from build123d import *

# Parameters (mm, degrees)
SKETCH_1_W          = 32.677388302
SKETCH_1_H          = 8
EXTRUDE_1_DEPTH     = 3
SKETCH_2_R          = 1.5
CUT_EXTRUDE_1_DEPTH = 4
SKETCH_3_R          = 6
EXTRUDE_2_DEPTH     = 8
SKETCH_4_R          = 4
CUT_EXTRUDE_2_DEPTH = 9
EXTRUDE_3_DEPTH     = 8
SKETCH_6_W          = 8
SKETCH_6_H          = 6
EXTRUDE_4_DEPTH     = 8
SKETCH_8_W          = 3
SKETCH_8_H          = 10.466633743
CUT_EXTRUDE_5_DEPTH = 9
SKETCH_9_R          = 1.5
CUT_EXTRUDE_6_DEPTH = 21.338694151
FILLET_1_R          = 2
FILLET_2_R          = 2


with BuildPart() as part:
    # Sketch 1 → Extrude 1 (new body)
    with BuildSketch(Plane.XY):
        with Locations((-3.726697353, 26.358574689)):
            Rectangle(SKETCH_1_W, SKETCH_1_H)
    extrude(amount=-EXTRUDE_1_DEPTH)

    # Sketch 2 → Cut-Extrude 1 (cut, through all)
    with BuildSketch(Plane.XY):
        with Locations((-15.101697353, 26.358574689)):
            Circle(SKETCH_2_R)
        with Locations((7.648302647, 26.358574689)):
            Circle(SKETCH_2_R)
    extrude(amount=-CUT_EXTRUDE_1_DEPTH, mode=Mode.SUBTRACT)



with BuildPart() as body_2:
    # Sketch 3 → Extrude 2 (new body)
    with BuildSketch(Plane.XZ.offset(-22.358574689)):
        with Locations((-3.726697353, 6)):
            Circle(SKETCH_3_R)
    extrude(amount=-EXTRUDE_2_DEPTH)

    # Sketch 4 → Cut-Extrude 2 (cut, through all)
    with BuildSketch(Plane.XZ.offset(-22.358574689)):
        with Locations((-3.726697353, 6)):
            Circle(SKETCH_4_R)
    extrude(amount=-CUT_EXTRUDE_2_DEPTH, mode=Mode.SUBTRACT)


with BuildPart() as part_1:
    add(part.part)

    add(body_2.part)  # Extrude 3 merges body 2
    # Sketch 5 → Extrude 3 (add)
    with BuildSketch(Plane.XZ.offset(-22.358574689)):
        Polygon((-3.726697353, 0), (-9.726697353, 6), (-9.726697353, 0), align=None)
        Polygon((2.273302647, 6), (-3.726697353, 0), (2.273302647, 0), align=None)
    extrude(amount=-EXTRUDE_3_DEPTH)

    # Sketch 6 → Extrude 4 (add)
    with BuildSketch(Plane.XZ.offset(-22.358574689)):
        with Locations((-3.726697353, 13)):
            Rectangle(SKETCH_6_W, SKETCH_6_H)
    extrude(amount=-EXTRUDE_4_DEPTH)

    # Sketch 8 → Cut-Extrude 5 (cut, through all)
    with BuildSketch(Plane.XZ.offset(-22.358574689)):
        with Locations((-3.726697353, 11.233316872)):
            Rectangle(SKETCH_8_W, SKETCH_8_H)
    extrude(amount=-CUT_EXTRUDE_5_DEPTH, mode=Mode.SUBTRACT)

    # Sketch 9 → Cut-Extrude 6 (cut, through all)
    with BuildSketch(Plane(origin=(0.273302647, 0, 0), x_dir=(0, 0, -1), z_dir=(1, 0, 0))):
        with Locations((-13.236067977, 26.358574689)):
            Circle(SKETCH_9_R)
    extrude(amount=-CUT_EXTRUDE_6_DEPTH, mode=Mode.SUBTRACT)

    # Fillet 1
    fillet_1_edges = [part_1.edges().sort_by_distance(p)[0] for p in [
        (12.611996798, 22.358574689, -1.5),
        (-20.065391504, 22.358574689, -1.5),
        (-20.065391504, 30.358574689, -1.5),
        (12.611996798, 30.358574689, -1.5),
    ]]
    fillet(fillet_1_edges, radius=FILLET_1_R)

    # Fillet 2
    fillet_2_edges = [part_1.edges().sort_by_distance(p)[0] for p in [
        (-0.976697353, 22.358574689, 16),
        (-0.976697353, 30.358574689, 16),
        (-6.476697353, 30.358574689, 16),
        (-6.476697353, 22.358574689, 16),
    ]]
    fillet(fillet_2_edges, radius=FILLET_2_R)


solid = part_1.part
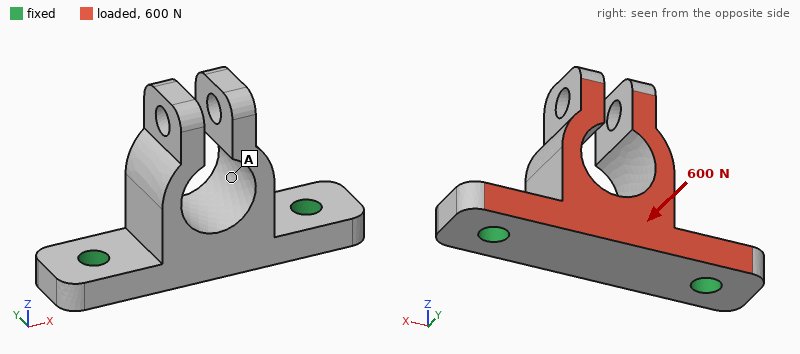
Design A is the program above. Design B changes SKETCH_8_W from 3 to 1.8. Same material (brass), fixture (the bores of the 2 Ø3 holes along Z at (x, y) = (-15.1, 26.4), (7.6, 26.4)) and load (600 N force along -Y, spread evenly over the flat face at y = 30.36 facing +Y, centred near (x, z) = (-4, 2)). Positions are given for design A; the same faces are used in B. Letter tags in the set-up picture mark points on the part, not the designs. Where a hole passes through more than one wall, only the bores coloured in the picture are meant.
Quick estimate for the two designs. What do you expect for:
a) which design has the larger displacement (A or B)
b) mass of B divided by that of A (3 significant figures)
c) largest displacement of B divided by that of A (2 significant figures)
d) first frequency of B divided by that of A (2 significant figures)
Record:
B
1.03
1.1
0.93
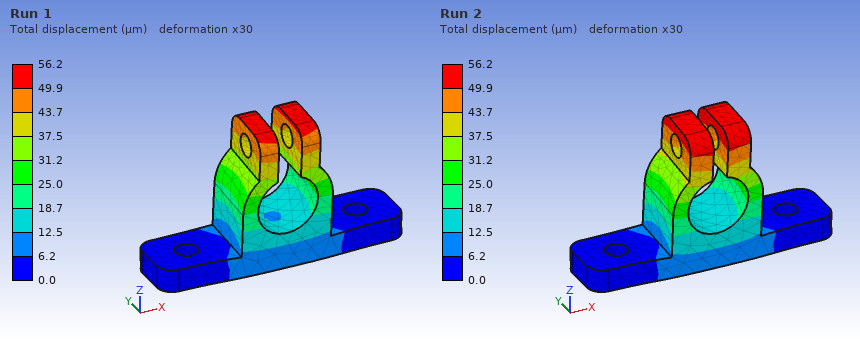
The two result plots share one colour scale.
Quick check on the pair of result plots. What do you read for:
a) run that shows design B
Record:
Run 2
